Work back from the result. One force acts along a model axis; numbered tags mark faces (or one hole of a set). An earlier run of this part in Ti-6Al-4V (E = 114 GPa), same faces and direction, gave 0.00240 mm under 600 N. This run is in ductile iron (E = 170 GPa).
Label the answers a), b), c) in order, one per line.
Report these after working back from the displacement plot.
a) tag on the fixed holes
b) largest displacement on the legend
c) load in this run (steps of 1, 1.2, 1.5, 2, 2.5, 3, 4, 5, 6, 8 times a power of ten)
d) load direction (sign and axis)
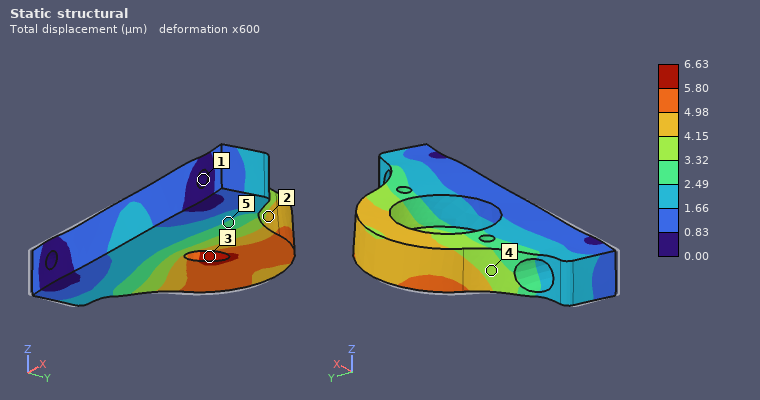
a) 1
b) 6.63 µm
c) 2.5 kN
d) +X
